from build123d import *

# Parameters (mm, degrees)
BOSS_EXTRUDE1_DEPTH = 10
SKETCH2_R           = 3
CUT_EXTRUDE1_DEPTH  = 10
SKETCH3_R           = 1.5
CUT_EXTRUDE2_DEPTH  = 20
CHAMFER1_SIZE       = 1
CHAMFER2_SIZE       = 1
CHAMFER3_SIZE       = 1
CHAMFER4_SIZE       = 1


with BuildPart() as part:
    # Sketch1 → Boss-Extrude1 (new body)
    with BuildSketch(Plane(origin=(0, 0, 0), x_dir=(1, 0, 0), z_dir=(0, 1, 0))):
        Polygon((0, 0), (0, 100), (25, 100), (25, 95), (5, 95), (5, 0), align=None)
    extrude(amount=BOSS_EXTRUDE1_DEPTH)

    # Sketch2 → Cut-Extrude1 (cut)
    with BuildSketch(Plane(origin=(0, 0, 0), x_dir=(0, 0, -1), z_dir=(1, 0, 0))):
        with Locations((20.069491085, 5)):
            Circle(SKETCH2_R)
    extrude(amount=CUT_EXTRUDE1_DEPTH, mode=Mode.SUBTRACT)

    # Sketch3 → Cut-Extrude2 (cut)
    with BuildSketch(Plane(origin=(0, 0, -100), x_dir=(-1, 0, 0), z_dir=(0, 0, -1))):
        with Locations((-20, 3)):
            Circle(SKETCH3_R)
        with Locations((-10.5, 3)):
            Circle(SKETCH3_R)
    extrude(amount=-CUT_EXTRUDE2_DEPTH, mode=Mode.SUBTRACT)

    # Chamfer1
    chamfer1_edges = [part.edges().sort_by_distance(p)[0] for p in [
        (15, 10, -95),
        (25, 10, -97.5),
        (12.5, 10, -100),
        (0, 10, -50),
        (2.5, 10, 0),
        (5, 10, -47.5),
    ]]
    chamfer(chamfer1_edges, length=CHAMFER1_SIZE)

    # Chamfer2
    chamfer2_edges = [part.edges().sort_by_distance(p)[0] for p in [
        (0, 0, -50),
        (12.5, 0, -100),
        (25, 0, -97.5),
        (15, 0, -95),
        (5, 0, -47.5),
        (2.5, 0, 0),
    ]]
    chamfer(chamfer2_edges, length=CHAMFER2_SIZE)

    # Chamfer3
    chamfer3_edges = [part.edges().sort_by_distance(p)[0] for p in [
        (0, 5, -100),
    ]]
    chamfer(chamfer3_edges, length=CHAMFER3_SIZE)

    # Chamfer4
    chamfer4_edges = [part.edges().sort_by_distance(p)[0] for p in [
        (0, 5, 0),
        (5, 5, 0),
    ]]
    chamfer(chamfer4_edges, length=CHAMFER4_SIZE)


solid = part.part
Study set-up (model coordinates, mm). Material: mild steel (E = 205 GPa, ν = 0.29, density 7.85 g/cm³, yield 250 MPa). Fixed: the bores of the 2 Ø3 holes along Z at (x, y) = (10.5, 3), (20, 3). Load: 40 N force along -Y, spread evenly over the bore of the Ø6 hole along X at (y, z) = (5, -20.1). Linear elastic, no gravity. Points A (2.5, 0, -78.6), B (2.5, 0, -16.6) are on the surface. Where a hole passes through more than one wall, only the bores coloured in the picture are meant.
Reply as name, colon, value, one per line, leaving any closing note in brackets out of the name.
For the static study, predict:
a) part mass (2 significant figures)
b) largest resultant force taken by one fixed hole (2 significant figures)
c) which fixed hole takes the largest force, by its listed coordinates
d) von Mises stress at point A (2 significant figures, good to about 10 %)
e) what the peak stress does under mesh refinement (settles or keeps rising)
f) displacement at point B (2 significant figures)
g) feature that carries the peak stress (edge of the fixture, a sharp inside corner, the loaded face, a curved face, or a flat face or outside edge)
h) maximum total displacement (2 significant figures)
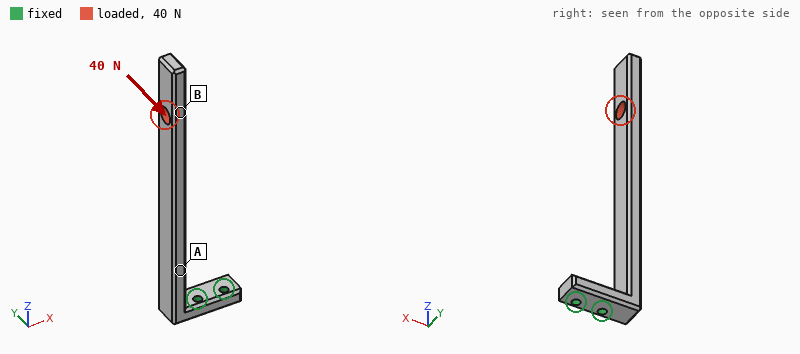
part mass: 43 g
largest resultant force taken by one fixed hole: 60 N
which fixed hole takes the largest force, by its listed coordinates: (10.5, 3)
von Mises stress at point A: 31 MPa
what the peak stress does under mesh refinement: keeps rising
displacement at point B: 0.16 mm
feature that carries the peak stress: edge of the fixture
maximum total displacement: 0.20 mm
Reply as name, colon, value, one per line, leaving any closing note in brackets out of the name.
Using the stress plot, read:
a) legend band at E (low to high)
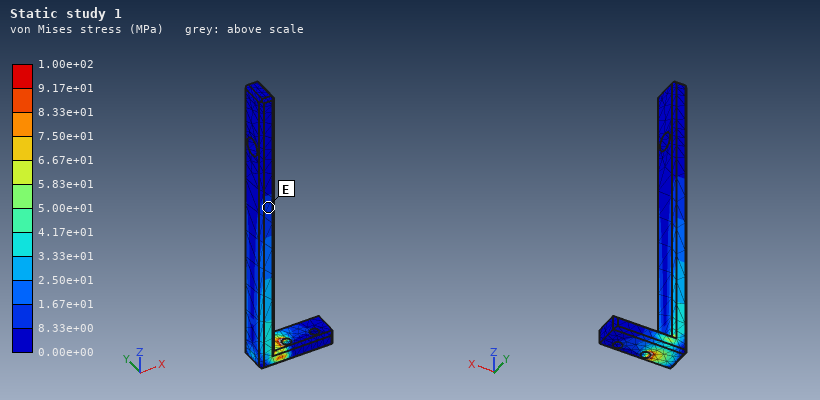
legend band at E: 8.33e+00 to 1.67e+01 MPa
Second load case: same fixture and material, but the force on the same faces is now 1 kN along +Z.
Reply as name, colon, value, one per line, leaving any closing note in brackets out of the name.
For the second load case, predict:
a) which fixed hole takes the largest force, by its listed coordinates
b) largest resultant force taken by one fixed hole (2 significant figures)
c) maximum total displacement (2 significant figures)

which fixed hole takes the largest force, by its listed coordinates: (10.5, 3)
largest resultant force taken by one fixed hole: 1.1 kN
maximum total displacement: 0.17 mm
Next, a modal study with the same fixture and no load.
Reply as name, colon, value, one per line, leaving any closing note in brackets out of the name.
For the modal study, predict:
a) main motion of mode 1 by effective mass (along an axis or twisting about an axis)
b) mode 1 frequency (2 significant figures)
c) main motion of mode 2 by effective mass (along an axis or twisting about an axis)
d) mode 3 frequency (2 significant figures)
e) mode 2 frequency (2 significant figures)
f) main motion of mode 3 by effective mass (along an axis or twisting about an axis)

main motion of mode 1 by effective mass: along X
mode 1 frequency: 390 Hz
main motion of mode 2 by effective mass: along Y
mode 3 frequency: 2300 Hz
mode 2 frequency: 630 Hz
main motion of mode 3 by effective mass: along X
